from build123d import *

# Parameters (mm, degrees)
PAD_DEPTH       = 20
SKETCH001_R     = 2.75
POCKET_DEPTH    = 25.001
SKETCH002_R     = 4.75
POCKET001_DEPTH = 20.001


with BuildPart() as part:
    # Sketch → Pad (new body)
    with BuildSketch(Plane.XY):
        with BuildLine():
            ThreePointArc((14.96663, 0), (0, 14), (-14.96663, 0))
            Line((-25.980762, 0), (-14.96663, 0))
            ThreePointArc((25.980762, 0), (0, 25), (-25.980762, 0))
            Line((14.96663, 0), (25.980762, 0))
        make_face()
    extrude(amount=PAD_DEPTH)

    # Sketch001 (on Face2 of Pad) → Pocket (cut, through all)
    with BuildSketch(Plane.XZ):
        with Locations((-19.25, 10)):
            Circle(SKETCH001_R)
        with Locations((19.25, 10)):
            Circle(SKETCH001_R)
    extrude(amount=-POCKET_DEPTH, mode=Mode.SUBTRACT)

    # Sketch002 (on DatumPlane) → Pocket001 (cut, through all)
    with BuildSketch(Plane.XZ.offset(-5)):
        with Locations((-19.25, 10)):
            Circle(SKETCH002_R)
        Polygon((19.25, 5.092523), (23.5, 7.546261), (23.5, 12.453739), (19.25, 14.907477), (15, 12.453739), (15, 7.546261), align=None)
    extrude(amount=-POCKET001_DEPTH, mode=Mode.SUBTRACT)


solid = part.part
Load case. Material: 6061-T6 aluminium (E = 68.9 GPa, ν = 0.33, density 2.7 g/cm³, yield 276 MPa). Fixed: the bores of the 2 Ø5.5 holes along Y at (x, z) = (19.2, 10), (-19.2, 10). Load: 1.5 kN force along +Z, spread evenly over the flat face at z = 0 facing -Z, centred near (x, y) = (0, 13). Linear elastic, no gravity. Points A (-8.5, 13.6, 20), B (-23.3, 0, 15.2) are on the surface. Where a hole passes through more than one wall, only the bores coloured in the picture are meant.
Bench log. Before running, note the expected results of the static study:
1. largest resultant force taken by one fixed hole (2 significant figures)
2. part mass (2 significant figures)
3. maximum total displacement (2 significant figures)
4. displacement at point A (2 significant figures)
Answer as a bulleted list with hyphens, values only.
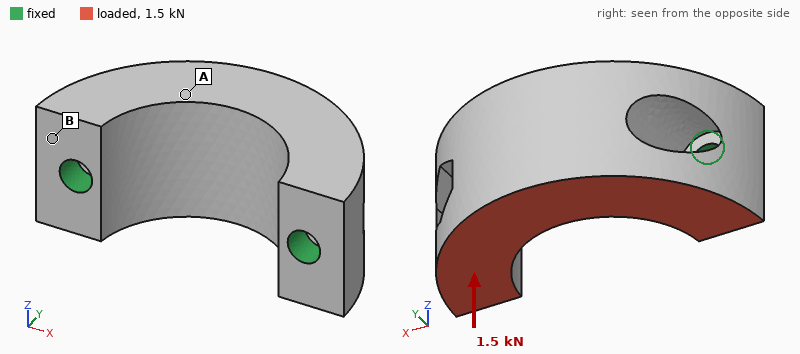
- 750 N
- 32 g
- 30 µm
- 18 µm
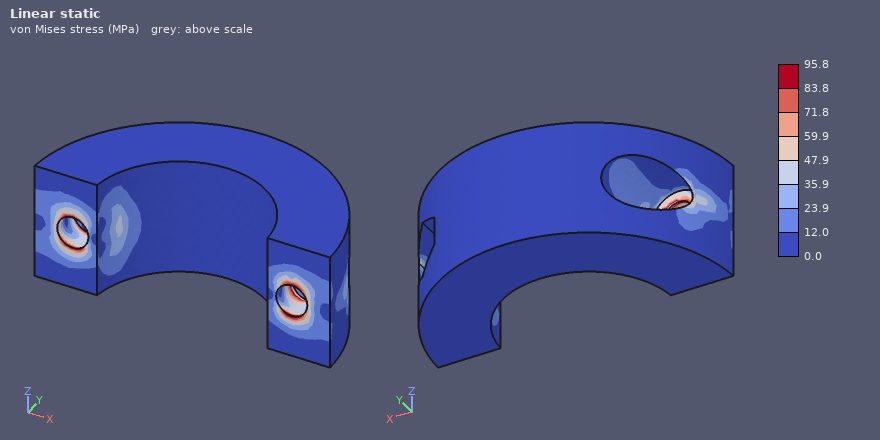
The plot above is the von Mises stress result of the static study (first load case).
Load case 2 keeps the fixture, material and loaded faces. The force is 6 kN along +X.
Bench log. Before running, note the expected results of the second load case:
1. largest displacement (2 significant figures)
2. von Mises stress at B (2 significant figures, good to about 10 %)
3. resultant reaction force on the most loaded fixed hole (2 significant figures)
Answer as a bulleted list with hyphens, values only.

- 41 µm
- 26 MPa
- 3.4 kN
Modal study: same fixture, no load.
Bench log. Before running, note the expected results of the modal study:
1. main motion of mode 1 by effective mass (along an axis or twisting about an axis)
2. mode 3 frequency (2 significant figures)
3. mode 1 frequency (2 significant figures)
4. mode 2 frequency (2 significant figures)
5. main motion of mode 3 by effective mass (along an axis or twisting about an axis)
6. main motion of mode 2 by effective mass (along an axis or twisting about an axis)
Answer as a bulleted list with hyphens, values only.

- along Z
- 19 kHz
- 7200 Hz
- 16 kHz
- twisting about Y
- along X
